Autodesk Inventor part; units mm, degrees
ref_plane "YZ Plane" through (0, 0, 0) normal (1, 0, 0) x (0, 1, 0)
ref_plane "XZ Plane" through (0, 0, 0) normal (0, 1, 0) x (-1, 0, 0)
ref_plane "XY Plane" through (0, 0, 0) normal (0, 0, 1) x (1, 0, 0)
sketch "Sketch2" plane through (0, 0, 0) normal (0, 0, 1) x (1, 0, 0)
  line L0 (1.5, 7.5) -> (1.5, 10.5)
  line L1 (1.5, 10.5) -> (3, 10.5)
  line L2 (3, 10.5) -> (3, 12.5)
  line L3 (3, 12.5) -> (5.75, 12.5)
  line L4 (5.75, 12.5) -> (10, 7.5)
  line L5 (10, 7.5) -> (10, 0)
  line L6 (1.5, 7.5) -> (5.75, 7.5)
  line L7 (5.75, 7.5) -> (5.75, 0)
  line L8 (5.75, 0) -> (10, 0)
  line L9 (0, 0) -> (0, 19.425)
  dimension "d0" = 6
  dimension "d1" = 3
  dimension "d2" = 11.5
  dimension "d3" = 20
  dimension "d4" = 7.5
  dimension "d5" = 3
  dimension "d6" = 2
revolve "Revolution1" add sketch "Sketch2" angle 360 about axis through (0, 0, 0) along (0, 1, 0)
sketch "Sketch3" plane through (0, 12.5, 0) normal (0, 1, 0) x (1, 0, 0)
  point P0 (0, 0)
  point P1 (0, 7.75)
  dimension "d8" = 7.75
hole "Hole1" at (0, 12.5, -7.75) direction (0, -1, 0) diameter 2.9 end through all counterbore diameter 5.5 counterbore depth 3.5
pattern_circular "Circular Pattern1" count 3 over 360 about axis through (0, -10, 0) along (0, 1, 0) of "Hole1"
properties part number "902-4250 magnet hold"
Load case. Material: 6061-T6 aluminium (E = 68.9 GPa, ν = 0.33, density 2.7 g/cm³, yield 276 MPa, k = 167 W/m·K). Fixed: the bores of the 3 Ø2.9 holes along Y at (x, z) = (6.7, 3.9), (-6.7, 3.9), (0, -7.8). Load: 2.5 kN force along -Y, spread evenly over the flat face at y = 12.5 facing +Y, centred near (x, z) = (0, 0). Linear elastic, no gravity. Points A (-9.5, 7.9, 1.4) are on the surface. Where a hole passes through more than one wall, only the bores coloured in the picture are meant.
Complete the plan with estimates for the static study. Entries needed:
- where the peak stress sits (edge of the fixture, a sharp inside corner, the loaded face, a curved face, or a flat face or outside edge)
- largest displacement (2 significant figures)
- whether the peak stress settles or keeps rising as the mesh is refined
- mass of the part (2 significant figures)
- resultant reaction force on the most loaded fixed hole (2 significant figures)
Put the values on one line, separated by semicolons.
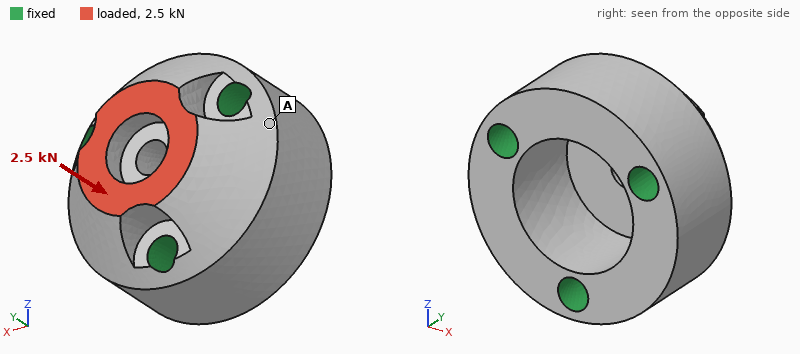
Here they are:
edge of the fixture; 6.3 µm; keeps rising; 6.0 g; 880 N
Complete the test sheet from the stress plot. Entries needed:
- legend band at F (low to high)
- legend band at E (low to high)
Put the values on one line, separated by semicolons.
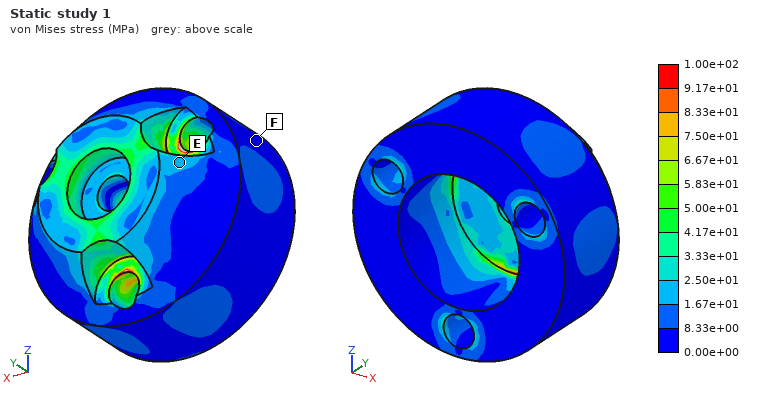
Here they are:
0.00e+00 to 8.33e+00 MPa; 1.67e+01 to 2.50e+01 MPa
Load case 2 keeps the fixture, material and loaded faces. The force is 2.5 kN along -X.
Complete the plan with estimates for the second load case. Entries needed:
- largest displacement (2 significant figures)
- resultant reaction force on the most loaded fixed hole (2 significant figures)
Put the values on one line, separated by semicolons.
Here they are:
12 µm; 1.2 kN
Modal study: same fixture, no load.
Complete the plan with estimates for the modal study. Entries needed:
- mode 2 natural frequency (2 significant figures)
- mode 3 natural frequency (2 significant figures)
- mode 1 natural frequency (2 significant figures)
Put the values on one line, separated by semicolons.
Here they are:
81 kHz; 82 kHz; 81 kHz
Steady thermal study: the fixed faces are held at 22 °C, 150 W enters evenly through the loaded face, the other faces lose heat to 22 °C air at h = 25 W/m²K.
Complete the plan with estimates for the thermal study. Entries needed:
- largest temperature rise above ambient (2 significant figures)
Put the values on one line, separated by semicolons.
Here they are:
65 K
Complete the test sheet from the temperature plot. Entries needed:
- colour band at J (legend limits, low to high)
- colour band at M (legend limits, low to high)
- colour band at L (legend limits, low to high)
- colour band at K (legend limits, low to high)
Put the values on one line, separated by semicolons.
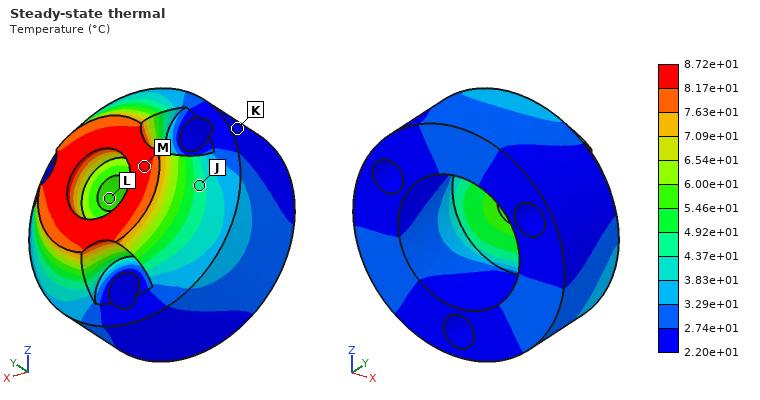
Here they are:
4.37e+01 to 4.92e+01 °C; 8.17e+01 to 8.72e+01 °C; 5.46e+01 to 6.00e+01 °C; 2.20e+01 to 2.74e+01 °C
